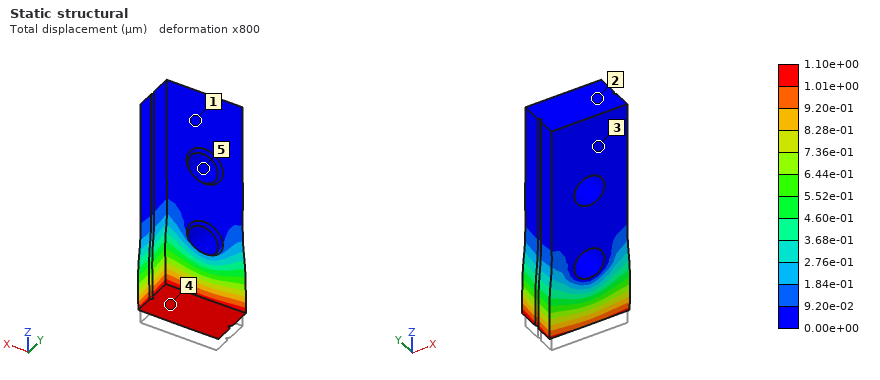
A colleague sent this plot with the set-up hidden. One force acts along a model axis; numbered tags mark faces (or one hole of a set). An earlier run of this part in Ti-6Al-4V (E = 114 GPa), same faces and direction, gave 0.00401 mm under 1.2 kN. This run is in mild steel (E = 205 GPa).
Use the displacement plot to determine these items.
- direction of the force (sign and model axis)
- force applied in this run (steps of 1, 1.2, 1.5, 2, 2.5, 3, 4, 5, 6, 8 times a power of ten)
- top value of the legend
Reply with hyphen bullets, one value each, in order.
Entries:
- +Z
- 600 N
- 1.10e+00 µm
